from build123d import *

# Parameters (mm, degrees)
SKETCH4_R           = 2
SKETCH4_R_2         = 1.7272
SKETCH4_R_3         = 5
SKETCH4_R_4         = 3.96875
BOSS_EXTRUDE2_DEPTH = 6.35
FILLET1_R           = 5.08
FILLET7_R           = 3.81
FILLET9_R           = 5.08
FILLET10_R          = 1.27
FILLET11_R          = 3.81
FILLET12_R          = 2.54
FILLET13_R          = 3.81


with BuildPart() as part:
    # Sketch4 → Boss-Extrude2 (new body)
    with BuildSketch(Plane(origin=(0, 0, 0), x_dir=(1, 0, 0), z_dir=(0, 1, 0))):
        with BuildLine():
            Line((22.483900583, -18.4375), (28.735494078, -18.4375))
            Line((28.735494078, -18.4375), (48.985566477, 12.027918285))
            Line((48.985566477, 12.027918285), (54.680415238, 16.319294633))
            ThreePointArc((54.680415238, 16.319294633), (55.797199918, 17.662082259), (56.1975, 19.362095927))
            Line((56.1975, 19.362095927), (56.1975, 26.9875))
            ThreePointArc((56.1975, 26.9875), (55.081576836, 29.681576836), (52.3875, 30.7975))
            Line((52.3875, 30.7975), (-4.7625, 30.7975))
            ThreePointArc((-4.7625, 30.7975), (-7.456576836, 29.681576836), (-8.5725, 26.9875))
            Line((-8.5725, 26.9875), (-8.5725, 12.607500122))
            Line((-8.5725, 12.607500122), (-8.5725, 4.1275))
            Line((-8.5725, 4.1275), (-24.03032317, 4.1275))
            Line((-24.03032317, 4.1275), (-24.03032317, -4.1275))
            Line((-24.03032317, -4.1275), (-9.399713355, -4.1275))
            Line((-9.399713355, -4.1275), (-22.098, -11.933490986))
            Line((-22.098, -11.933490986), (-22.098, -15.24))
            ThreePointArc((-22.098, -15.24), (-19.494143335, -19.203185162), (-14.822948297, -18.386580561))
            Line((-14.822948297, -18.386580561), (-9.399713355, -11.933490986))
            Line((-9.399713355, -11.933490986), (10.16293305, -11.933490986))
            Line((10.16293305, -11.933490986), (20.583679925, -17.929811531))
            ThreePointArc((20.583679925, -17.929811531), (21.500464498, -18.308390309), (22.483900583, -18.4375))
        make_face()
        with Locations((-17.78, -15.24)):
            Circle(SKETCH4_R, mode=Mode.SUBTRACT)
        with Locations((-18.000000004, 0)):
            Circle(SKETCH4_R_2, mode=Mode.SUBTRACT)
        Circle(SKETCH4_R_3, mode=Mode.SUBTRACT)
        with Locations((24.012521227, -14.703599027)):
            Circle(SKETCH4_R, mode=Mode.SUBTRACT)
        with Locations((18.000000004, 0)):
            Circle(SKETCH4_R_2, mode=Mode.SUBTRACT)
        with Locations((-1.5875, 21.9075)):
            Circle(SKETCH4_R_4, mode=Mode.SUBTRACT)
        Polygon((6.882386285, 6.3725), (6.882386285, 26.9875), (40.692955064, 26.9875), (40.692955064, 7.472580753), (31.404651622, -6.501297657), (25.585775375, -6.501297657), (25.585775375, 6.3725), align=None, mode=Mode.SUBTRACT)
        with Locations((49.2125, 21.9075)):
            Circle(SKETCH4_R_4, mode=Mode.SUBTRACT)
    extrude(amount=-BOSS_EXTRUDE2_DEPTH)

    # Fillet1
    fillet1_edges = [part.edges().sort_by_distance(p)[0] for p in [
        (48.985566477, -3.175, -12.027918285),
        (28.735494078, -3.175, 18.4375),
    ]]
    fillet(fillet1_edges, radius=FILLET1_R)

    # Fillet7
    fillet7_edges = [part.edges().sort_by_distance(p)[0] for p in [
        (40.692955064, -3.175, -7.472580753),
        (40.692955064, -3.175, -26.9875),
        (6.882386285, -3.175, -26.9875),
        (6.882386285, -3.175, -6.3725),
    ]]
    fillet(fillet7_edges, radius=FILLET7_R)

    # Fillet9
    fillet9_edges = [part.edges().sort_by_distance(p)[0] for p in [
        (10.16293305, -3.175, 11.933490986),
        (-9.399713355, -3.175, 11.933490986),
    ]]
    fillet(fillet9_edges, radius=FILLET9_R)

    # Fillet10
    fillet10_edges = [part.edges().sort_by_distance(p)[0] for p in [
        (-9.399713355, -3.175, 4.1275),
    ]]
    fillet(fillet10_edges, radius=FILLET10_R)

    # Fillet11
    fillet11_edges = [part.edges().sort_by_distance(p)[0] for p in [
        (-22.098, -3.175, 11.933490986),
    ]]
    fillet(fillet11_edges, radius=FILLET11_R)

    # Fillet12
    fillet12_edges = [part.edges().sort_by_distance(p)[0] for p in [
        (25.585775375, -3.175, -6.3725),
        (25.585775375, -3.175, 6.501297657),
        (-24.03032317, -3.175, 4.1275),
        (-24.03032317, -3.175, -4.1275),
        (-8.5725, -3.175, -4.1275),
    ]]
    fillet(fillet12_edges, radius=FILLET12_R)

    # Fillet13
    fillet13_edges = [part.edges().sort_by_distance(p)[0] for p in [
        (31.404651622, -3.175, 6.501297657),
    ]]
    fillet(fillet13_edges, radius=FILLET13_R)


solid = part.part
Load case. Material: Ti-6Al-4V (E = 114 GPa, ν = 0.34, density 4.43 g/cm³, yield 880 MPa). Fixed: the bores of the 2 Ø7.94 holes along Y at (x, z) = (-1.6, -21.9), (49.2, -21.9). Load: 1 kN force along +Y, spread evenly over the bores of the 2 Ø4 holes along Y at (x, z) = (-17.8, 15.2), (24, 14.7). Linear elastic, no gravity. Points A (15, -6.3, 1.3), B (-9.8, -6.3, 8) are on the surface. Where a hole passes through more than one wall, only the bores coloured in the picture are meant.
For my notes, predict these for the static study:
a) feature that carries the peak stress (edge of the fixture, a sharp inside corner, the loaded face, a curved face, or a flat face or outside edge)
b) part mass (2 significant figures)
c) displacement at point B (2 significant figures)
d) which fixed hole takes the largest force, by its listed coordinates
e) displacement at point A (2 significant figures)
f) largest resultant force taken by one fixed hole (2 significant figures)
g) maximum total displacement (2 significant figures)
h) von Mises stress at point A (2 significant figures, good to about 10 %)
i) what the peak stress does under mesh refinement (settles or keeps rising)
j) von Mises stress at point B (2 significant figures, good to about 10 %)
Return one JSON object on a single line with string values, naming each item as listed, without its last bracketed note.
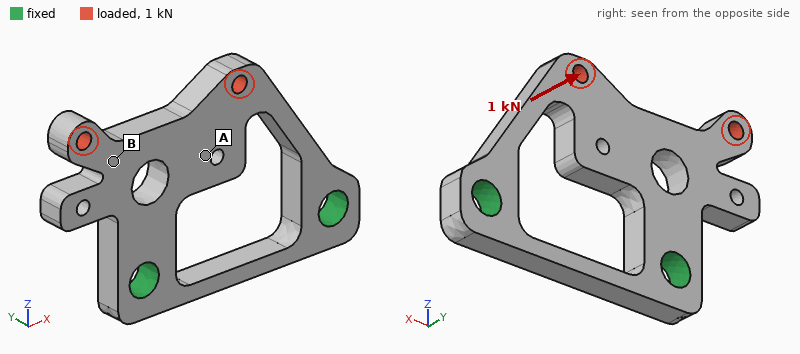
{"feature that carries the peak stress": "edge of the fixture", "part mass": "48 g", "displacement at point B": "0.23 mm", "which fixed hole takes the largest force, by its listed coordinates": "(-1.6, -21.9)", "displacement at point A": "0.12 mm", "largest resultant force taken by one fixed hole": "800 N", "maximum total displacement": "0.42 mm", "von Mises stress at point A": "33 MPa", "what the peak stress does under mesh refinement": "keeps rising", "von Mises stress at point B": "87 MPa"}
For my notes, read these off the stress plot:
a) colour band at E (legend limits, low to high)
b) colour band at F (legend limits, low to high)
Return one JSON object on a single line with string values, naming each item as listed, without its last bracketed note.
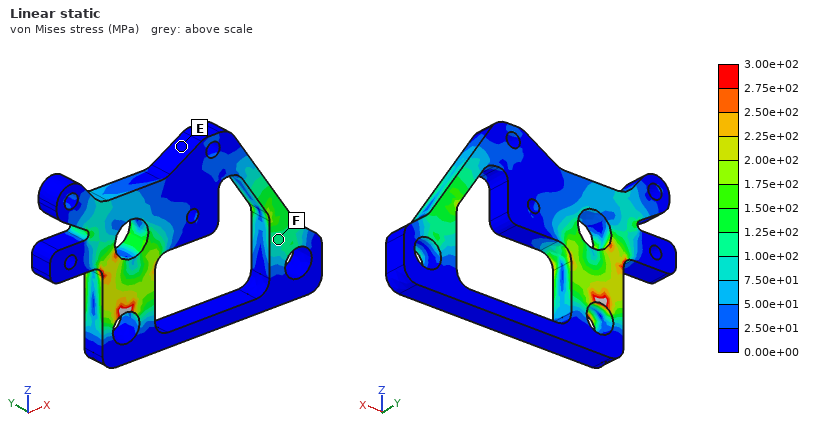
{"colour band at E": "0.00e+00 to 2.50e+01 MPa", "colour band at F": "1.00e+02 to 1.25e+02 MPa"}
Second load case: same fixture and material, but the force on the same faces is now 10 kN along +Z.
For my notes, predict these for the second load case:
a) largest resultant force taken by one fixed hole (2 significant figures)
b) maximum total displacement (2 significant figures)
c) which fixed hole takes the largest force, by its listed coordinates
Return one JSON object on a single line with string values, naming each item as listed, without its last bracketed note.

{"largest resultant force taken by one fixed hole": "8.8 kN", "maximum total displacement": "0.26 mm", "which fixed hole takes the largest force, by its listed coordinates": "(-1.6, -21.9)"}
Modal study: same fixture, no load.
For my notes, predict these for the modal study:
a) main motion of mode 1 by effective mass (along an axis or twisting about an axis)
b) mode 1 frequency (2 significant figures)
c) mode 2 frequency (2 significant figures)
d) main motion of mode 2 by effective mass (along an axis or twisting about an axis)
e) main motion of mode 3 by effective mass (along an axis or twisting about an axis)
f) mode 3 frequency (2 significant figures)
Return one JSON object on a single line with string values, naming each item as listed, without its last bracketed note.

{"main motion of mode 1 by effective mass": "along Y", "mode 1 frequency": "2800 Hz", "mode 2 frequency": "4200 Hz", "main motion of mode 2 by effective mass": "twisting about Z", "main motion of mode 3 by effective mass": "along X", "mode 3 frequency": "9200 Hz"}
